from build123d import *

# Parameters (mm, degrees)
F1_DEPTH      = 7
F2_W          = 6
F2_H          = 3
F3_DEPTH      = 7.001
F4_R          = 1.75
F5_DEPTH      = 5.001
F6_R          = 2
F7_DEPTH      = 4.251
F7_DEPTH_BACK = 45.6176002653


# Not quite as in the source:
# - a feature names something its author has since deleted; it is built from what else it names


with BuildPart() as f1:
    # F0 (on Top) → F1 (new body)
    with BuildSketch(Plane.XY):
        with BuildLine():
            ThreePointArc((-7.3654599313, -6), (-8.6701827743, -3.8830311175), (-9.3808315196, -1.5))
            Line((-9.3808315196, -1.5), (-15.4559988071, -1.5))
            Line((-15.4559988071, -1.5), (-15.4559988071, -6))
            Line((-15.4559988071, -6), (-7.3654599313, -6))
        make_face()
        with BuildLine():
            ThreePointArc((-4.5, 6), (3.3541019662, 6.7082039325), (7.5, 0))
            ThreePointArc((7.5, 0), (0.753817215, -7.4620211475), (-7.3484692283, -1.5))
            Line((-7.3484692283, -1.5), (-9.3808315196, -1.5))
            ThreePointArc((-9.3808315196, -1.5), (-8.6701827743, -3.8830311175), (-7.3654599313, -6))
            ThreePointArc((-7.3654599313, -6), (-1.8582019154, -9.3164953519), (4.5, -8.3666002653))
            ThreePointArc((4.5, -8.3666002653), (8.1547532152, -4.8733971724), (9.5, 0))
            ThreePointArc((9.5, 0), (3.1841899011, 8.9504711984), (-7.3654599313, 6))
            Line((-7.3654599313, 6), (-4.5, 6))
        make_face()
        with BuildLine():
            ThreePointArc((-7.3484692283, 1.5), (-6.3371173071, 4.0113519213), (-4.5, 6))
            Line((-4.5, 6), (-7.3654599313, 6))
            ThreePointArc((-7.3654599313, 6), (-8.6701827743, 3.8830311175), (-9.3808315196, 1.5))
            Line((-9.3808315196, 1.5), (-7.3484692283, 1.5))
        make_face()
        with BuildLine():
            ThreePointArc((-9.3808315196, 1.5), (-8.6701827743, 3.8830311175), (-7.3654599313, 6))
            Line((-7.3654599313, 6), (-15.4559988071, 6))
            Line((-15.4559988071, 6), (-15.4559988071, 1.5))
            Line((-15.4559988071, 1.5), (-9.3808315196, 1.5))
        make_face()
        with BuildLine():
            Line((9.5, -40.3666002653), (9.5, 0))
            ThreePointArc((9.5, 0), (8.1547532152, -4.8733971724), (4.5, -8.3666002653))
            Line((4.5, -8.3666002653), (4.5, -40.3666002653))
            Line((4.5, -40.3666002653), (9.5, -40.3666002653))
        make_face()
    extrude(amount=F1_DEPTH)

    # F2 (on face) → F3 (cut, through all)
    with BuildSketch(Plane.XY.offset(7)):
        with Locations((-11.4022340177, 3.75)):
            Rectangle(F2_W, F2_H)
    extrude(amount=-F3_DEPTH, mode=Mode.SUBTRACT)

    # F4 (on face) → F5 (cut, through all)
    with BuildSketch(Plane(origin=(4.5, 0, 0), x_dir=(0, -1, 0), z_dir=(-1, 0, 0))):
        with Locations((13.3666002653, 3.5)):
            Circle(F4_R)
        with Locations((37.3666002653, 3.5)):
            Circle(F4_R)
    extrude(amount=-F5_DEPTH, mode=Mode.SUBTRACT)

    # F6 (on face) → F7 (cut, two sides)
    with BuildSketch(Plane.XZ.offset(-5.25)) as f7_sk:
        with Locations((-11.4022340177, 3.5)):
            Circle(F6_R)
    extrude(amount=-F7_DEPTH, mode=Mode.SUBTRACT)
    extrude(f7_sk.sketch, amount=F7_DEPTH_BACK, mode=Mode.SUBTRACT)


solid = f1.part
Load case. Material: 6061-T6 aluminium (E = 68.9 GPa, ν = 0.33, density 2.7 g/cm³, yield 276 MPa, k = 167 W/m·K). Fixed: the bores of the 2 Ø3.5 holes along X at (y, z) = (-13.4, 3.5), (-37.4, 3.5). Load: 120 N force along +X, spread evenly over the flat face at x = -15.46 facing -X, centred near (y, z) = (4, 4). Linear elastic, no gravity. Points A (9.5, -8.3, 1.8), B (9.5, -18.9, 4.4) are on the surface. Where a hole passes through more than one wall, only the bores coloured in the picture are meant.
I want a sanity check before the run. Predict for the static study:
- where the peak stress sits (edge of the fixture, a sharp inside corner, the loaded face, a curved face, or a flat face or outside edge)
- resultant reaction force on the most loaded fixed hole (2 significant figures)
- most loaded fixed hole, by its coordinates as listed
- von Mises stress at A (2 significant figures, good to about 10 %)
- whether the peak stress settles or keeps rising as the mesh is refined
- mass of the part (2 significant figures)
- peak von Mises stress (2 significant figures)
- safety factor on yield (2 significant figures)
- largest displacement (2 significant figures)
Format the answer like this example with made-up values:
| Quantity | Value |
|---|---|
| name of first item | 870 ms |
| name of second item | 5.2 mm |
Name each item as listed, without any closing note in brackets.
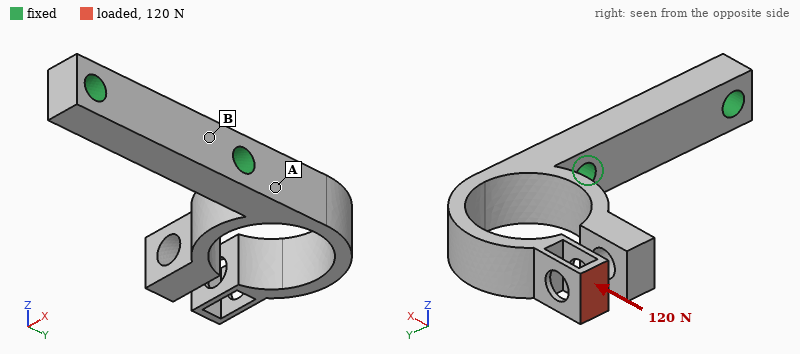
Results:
| Quantity | Value |
|---|---|
| where the peak stress sits | a curved face |
| resultant reaction force on the most loaded fixed hole | 120 N |
| most loaded fixed hole, by its coordinates as listed | (-13.4, 3.5) |
| von Mises stress at A | 51 MPa |
| whether the peak stress settles or keeps rising as the mesh is refined | settles |
| mass of the part | 5.5 g |
| peak von Mises stress | 140 MPa |
| safety factor on yield | 2.0 |
| largest displacement | 0.20 mm |
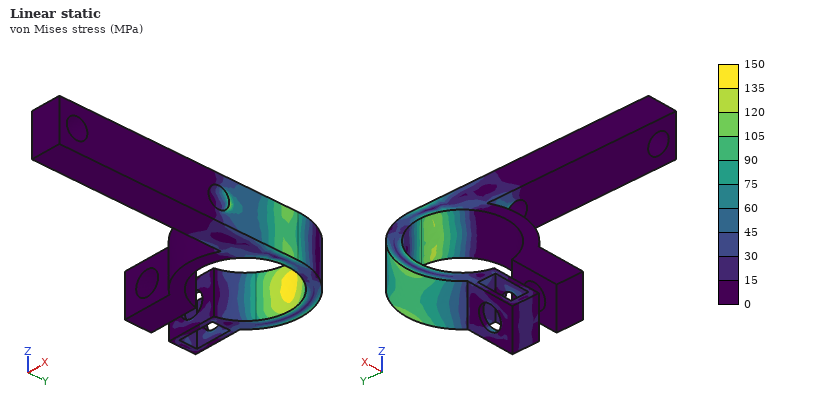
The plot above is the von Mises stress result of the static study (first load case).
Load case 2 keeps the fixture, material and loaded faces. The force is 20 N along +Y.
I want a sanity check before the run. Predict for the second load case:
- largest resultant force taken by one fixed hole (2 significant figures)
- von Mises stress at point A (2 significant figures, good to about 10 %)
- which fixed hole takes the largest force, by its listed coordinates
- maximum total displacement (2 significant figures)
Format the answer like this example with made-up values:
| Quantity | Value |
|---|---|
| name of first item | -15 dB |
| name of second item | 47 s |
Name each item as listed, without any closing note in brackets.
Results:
| Quantity | Value |
|---|---|
| largest resultant force taken by one fixed hole | 20 N |
| von Mises stress at point A | 16 MPa |
| which fixed hole takes the largest force, by its listed coordinates | (-13.4, 3.5) |
| maximum total displacement | 0.59 mm |
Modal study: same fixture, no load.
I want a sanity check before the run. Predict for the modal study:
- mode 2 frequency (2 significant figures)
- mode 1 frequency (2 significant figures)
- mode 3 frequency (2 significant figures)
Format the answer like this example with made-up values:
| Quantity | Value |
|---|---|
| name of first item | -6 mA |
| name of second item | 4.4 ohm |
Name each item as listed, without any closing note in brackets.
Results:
| Quantity | Value |
|---|---|
| mode 2 frequency | 2300 Hz |
| mode 1 frequency | 1700 Hz |
| mode 3 frequency | 2700 Hz |
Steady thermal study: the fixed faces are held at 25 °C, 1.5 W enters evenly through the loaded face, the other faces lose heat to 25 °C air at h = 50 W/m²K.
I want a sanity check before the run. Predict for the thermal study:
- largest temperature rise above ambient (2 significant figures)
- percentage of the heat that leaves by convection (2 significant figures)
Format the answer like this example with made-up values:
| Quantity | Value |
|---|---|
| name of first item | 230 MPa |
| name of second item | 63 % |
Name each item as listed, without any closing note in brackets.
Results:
| Quantity | Value |
|---|---|
| largest temperature rise above ambient | 24 K |
| percentage of the heat that leaves by convection | 30 % |
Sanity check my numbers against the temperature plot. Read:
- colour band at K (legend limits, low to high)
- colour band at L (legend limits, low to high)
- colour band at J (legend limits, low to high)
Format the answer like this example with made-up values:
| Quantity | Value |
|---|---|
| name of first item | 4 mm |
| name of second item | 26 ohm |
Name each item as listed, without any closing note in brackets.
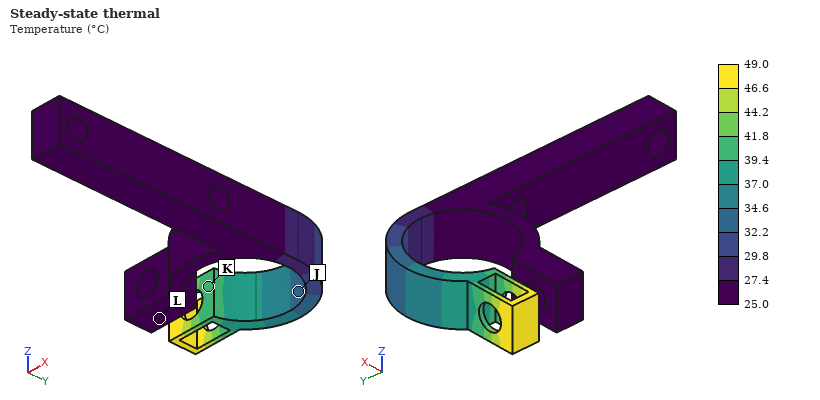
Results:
| Quantity | Value |
|---|---|
| colour band at K | 39.4 to 41.8 °C |
| colour band at L | 25.0 to 27.4 °C |
| colour band at J | 32.2 to 34.6 °C |
